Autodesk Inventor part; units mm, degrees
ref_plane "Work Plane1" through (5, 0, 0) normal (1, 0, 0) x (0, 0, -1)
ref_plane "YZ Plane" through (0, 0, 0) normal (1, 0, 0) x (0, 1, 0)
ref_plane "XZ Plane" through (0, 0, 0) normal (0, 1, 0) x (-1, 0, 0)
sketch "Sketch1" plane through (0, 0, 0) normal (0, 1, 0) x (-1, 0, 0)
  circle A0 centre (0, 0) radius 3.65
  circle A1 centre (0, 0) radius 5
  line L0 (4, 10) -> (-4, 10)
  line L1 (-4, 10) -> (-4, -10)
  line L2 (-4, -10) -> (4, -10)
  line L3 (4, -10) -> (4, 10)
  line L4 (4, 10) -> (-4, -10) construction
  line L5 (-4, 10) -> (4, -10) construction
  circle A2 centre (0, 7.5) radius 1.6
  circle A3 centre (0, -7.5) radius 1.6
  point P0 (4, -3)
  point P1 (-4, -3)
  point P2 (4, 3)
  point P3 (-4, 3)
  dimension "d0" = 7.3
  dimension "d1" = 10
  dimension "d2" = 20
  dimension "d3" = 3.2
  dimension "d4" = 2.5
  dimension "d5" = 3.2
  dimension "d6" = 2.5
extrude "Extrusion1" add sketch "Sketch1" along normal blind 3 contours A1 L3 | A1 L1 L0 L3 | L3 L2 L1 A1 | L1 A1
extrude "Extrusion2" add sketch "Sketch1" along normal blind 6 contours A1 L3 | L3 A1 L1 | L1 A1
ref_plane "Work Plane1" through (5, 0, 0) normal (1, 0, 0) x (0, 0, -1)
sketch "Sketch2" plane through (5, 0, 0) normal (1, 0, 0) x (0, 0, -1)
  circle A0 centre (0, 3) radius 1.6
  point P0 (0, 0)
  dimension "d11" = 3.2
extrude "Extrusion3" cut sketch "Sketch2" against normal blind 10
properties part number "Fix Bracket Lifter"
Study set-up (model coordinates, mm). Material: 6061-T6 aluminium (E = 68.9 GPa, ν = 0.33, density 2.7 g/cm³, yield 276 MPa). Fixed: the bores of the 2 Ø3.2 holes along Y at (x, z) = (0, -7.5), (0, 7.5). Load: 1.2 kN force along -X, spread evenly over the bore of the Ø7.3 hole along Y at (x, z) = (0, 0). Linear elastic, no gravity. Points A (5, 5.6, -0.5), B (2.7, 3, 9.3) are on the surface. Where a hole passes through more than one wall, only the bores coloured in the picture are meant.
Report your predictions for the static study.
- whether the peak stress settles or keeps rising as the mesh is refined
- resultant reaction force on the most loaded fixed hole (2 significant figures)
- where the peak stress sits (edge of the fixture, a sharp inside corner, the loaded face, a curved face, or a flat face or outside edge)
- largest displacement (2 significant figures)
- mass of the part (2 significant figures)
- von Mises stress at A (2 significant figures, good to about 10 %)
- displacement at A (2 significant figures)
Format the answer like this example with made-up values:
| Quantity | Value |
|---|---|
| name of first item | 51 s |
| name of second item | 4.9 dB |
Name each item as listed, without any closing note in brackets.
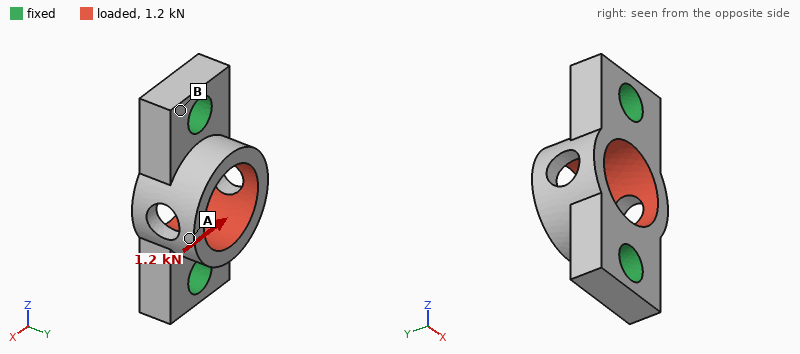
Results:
| Quantity | Value |
|---|---|
| whether the peak stress settles or keeps rising as the mesh is refined | keeps rising |
| resultant reaction force on the most loaded fixed hole | 600 N |
| where the peak stress sits | edge of the fixture |
| largest displacement | 19 µm |
| mass of the part | 1.1 g |
| von Mises stress at A | 39 MPa |
| displacement at A | 18 µm |
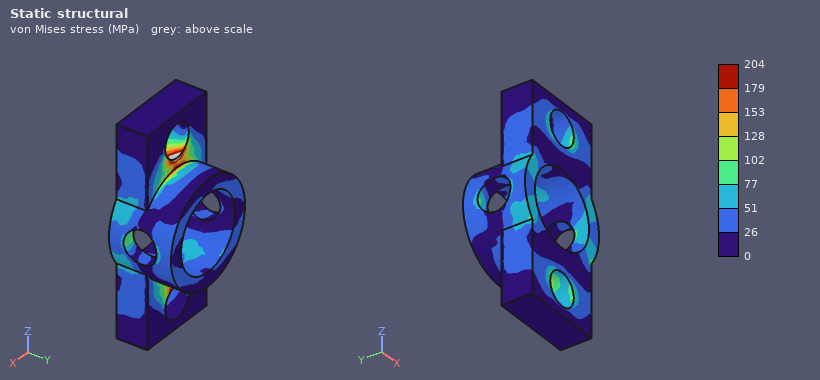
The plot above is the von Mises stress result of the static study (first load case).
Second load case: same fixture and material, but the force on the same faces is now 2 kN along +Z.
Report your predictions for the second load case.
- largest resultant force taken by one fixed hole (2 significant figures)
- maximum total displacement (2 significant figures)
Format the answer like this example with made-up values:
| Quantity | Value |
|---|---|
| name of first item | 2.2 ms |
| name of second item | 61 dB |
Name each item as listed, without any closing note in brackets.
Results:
| Quantity | Value |
|---|---|
| largest resultant force taken by one fixed hole | 1.0 kN |
| maximum total displacement | 14 µm |
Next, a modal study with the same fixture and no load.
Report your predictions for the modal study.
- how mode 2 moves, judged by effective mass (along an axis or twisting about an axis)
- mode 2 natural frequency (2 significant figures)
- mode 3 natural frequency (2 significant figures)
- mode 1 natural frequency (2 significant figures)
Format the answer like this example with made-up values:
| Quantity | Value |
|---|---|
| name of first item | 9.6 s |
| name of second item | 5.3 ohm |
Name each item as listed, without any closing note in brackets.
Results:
| Quantity | Value |
|---|---|
| how mode 2 moves, judged by effective mass | along Y |
| mode 2 natural frequency | 63 kHz |
| mode 3 natural frequency | 79 kHz |
| mode 1 natural frequency | 53 kHz |
